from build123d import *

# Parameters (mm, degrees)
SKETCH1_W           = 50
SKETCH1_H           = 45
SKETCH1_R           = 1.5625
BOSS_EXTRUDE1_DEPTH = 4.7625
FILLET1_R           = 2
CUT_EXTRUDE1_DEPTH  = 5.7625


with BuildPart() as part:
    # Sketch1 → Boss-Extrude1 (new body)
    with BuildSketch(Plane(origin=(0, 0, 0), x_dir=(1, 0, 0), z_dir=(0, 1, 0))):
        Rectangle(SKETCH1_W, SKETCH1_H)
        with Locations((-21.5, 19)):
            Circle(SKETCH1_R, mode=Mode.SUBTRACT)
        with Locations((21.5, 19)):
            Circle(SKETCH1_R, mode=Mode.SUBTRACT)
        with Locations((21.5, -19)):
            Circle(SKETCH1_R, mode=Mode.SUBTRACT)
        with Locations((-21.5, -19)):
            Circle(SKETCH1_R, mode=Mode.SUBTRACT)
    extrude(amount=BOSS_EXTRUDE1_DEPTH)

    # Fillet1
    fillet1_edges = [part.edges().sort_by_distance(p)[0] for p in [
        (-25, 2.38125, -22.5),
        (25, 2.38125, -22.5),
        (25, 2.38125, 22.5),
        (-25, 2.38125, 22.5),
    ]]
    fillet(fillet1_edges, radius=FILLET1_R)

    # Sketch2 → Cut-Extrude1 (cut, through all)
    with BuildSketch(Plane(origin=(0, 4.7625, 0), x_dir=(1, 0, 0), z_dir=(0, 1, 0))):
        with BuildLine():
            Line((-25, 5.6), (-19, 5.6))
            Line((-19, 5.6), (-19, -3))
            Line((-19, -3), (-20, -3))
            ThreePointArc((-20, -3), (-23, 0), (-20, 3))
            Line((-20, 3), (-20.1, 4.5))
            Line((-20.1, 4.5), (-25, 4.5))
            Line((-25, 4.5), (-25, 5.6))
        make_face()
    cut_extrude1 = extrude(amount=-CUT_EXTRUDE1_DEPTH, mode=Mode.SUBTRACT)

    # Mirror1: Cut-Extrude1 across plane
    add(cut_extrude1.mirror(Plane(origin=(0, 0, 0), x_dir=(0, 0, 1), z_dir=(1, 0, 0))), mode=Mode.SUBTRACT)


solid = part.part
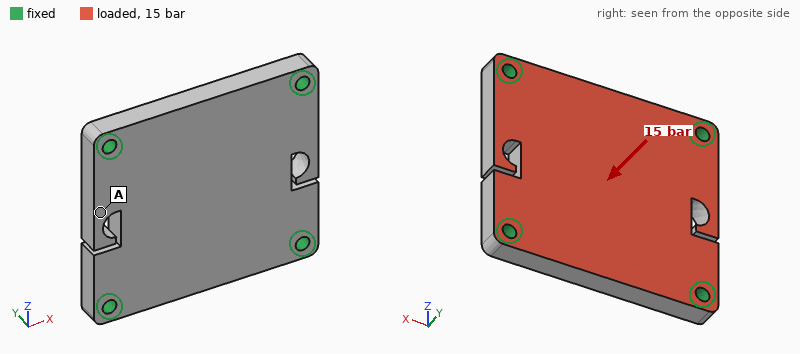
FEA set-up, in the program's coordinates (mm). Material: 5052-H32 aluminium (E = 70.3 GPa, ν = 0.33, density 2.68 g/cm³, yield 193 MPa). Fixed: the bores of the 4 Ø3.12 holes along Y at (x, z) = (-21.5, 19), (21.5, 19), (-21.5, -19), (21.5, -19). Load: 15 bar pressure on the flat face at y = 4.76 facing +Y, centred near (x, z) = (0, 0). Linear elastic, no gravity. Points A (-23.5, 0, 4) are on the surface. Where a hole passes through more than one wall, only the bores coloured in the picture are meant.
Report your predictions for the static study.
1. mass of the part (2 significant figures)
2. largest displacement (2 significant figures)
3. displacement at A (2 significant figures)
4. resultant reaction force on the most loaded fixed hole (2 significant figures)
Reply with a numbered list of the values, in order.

1. 28 g
2. 52 µm
3. 24 µm
4. 820 N
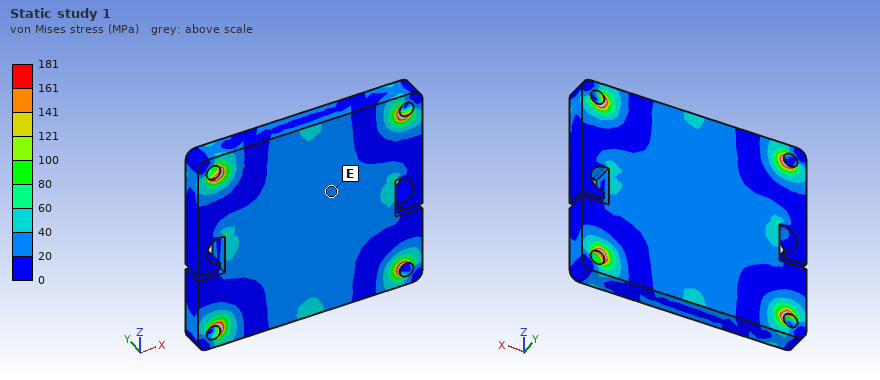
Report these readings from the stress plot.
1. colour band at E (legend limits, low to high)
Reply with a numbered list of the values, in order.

1. 20 to 40 MPa
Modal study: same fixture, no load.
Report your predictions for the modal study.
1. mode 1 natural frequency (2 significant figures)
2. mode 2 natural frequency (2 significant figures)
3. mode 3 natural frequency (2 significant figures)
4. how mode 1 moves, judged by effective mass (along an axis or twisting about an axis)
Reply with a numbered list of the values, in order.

1. 9000 Hz
2. 14 kHz
3. 14 kHz
4. along Y
